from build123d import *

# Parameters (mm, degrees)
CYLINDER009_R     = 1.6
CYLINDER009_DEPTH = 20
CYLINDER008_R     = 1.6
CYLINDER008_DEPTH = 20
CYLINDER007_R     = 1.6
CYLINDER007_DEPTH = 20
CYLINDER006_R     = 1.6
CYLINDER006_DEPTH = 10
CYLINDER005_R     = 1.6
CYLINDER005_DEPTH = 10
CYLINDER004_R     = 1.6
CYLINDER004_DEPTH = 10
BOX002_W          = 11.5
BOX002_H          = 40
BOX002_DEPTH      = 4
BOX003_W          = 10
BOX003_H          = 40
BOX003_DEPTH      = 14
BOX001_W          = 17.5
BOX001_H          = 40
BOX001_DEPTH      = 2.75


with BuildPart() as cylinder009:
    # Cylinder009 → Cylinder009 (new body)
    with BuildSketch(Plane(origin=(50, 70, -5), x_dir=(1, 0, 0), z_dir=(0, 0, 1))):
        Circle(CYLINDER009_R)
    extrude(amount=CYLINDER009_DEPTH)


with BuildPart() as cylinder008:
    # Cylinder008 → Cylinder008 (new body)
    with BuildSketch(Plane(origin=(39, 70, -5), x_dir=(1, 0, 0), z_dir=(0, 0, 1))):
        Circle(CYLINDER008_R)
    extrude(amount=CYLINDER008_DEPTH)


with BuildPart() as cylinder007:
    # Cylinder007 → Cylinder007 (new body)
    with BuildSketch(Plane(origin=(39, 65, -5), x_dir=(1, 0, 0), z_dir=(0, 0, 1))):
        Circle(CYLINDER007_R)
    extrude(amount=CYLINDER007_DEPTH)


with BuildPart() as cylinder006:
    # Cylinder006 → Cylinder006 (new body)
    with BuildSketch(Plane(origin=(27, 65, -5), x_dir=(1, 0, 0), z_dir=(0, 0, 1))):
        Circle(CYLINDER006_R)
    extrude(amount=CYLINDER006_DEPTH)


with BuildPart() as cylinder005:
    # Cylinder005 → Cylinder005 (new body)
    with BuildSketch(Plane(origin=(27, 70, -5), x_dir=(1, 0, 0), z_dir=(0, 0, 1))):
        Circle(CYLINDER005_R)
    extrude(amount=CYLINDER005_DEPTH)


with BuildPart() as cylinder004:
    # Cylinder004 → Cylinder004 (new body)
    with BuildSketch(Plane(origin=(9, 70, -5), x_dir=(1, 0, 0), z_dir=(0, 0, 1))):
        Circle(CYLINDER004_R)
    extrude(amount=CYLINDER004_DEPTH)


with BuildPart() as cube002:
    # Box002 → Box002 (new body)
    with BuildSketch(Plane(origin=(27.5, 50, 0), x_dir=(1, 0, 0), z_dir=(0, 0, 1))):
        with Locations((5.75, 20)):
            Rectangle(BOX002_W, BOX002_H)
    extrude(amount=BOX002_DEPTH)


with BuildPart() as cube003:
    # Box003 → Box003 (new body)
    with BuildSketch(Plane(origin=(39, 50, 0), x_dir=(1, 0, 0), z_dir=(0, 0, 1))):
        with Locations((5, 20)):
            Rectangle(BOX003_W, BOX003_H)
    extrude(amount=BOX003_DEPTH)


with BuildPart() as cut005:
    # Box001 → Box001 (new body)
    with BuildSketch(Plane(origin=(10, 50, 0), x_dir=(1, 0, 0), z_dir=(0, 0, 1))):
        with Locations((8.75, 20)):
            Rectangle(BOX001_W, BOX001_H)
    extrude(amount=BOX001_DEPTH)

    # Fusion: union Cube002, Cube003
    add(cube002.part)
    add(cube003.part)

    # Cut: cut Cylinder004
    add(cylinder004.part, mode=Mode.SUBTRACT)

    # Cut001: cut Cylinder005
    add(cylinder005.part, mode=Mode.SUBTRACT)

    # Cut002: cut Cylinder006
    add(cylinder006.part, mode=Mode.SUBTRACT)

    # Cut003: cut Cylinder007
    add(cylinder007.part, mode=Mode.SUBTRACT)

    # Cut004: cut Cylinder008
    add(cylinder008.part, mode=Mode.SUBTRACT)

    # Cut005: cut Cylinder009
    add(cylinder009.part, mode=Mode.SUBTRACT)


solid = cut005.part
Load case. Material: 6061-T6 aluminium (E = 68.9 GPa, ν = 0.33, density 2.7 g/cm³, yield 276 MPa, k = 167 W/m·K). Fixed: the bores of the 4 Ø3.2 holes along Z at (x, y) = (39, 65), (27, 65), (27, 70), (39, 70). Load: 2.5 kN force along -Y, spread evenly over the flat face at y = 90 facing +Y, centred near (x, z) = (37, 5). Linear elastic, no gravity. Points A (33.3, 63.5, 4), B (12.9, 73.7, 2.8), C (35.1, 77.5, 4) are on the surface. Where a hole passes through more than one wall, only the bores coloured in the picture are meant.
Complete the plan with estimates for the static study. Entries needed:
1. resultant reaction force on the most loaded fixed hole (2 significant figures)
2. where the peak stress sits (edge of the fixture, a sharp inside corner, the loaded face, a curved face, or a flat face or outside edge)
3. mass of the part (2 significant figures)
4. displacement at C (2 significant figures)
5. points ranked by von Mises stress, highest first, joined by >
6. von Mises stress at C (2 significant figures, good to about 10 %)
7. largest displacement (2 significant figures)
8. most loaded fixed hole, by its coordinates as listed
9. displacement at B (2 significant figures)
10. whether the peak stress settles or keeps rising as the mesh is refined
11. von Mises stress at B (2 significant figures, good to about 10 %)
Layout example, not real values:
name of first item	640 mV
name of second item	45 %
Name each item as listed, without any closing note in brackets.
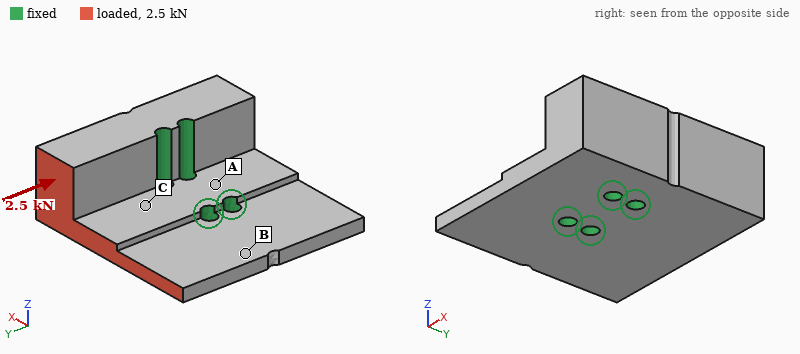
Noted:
resultant reaction force on the most loaded fixed hole	1.3 kN
where the peak stress sits	edge of the fixture
mass of the part	25 g
displacement at C	1.5 µm
points ranked by von Mises stress, highest first, joined by >	C > B > A
von Mises stress at C	13 MPa
largest displacement	6.9 µm
most loaded fixed hole, by its coordinates as listed	(39, 70)
displacement at B	3.6 µm
whether the peak stress settles or keeps rising as the mesh is refined	keeps rising
von Mises stress at B	7.4 MPa
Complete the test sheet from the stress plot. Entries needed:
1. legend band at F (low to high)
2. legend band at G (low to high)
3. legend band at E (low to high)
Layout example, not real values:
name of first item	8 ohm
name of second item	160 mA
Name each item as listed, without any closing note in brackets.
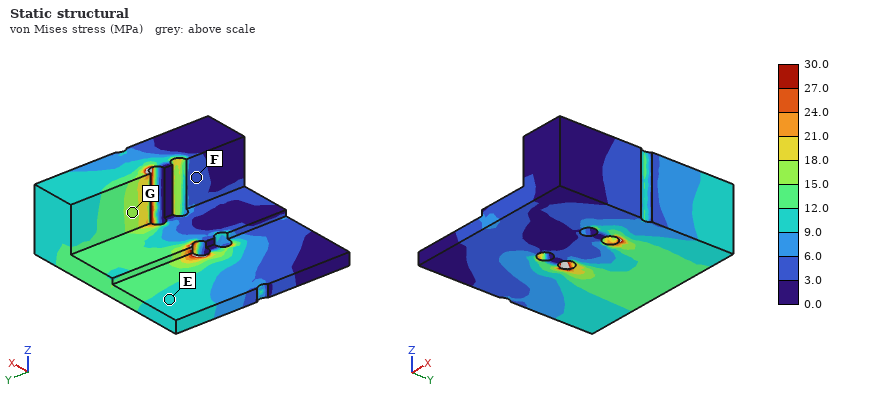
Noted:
legend band at F	3.0 to 6.0 MPa
legend band at G	15.0 to 18.0 MPa
legend band at E	9.0 to 12.0 MPa
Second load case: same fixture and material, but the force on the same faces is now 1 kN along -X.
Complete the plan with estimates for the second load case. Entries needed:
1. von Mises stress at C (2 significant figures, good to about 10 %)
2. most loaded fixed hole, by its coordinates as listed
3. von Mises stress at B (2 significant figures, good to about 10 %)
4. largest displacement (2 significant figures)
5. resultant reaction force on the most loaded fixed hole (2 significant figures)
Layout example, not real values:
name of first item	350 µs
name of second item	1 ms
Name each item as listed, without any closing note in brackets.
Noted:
von Mises stress at C	23 MPa
most loaded fixed hole, by its coordinates as listed	(39, 70)
von Mises stress at B	8.1 MPa
largest displacement	20 µm
resultant reaction force on the most loaded fixed hole	1.3 kN
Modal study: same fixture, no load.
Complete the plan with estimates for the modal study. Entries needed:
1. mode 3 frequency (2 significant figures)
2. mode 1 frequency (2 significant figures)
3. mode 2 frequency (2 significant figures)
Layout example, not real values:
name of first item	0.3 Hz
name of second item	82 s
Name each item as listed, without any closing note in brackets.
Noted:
mode 3 frequency	14 kHz
mode 1 frequency	6500 Hz
mode 2 frequency	7900 Hz
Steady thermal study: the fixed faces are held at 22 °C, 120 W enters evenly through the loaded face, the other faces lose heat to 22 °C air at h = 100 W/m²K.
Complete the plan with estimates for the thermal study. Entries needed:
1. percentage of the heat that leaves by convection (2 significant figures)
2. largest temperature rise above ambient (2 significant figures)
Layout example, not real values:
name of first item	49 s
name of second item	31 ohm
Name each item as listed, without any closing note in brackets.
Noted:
percentage of the heat that leaves by convection	7.0 %
largest temperature rise above ambient	67 K
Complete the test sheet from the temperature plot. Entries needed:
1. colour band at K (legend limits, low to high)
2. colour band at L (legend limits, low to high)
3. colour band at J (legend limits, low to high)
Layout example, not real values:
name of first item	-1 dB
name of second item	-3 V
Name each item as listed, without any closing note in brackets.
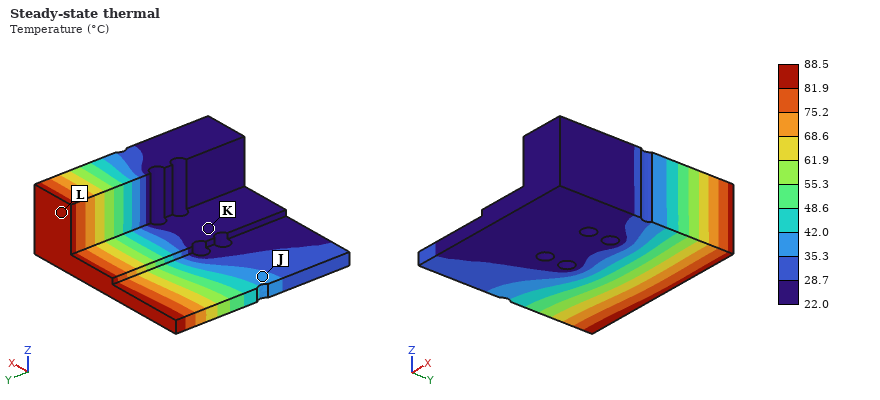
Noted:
colour band at K	22.0 to 28.7 °C
colour band at L	81.9 to 88.5 °C
colour band at J	35.3 to 42.0 °C
